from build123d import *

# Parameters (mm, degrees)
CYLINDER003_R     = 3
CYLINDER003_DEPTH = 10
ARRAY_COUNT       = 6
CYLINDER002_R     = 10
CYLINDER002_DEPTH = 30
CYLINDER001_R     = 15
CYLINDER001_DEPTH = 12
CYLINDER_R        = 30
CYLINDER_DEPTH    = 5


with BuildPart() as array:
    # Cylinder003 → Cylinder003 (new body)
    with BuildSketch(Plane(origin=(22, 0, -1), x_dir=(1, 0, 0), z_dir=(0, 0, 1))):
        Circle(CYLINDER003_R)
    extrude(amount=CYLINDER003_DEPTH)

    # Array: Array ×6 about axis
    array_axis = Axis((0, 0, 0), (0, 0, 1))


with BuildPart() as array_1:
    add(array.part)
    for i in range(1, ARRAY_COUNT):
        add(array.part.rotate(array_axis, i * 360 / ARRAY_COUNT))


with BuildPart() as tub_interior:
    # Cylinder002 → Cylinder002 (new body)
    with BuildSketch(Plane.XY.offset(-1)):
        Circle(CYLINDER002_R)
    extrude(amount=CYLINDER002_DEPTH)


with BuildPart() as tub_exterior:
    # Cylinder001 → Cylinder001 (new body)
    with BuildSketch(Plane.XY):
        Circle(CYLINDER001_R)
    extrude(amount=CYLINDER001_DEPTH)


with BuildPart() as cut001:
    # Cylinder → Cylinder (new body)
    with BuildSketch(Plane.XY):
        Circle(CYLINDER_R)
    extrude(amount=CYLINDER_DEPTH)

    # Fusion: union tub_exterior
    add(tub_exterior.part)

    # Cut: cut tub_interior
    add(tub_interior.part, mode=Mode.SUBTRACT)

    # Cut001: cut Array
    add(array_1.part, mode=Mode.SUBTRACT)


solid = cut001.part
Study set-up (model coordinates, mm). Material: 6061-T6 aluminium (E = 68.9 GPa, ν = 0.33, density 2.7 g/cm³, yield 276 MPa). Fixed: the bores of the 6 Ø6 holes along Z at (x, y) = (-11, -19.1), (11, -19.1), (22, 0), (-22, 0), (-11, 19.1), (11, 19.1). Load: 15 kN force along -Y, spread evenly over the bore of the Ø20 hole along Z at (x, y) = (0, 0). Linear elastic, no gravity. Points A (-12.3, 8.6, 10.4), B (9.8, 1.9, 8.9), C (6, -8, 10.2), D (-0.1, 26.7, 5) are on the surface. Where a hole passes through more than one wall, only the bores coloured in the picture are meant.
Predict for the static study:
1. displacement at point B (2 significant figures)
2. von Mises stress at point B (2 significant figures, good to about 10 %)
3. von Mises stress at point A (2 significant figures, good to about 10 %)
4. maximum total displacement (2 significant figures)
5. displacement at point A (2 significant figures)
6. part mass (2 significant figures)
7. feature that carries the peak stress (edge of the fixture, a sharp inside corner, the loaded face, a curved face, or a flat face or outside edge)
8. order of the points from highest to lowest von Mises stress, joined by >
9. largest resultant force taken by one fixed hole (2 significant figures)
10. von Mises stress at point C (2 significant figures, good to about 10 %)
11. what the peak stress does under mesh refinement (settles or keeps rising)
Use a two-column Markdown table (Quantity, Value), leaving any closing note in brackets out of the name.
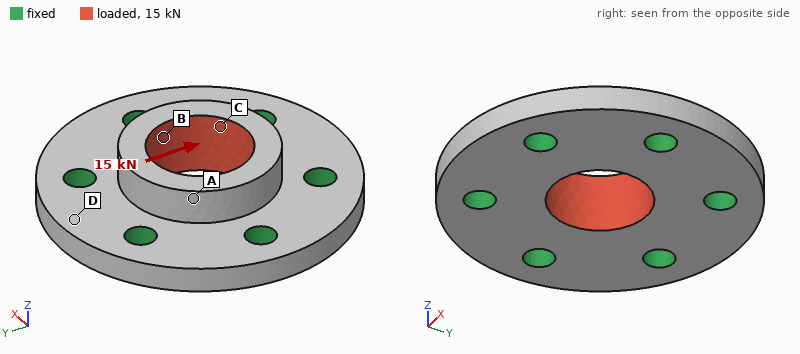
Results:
| Quantity | Value |
|---|---|
| displacement at point B | 13 µm |
| von Mises stress at point B | 57 MPa |
| von Mises stress at point A | 18 MPa |
| maximum total displacement | 21 µm |
| displacement at point A | 13 µm |
| part mass | 39 g |
| feature that carries the peak stress | edge of the fixture |
| order of the points from highest to lowest von Mises stress, joined by > | B > C > A > D |
| largest resultant force taken by one fixed hole | 3.2 kN |
| von Mises stress at point C | 46 MPa |
| what the peak stress does under mesh refinement | keeps rising |
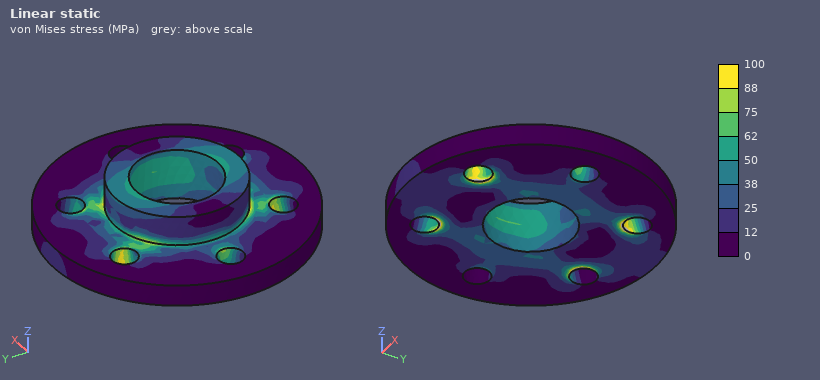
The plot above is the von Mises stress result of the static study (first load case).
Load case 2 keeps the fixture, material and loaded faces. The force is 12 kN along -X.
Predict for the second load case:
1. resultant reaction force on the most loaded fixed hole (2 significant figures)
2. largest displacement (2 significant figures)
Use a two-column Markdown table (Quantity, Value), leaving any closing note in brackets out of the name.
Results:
| Quantity | Value |
|---|---|
| resultant reaction force on the most loaded fixed hole | 2.9 kN |
| largest displacement | 17 µm |
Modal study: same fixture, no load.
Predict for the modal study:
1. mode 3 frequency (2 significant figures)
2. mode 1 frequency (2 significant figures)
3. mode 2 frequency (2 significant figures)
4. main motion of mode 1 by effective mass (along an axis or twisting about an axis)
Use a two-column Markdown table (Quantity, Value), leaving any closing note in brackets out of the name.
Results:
| Quantity | Value |
|---|---|
| mode 3 frequency | 36 kHz |
| mode 1 frequency | 32 kHz |
| mode 2 frequency | 35 kHz |
| main motion of mode 1 by effective mass | along Z |
